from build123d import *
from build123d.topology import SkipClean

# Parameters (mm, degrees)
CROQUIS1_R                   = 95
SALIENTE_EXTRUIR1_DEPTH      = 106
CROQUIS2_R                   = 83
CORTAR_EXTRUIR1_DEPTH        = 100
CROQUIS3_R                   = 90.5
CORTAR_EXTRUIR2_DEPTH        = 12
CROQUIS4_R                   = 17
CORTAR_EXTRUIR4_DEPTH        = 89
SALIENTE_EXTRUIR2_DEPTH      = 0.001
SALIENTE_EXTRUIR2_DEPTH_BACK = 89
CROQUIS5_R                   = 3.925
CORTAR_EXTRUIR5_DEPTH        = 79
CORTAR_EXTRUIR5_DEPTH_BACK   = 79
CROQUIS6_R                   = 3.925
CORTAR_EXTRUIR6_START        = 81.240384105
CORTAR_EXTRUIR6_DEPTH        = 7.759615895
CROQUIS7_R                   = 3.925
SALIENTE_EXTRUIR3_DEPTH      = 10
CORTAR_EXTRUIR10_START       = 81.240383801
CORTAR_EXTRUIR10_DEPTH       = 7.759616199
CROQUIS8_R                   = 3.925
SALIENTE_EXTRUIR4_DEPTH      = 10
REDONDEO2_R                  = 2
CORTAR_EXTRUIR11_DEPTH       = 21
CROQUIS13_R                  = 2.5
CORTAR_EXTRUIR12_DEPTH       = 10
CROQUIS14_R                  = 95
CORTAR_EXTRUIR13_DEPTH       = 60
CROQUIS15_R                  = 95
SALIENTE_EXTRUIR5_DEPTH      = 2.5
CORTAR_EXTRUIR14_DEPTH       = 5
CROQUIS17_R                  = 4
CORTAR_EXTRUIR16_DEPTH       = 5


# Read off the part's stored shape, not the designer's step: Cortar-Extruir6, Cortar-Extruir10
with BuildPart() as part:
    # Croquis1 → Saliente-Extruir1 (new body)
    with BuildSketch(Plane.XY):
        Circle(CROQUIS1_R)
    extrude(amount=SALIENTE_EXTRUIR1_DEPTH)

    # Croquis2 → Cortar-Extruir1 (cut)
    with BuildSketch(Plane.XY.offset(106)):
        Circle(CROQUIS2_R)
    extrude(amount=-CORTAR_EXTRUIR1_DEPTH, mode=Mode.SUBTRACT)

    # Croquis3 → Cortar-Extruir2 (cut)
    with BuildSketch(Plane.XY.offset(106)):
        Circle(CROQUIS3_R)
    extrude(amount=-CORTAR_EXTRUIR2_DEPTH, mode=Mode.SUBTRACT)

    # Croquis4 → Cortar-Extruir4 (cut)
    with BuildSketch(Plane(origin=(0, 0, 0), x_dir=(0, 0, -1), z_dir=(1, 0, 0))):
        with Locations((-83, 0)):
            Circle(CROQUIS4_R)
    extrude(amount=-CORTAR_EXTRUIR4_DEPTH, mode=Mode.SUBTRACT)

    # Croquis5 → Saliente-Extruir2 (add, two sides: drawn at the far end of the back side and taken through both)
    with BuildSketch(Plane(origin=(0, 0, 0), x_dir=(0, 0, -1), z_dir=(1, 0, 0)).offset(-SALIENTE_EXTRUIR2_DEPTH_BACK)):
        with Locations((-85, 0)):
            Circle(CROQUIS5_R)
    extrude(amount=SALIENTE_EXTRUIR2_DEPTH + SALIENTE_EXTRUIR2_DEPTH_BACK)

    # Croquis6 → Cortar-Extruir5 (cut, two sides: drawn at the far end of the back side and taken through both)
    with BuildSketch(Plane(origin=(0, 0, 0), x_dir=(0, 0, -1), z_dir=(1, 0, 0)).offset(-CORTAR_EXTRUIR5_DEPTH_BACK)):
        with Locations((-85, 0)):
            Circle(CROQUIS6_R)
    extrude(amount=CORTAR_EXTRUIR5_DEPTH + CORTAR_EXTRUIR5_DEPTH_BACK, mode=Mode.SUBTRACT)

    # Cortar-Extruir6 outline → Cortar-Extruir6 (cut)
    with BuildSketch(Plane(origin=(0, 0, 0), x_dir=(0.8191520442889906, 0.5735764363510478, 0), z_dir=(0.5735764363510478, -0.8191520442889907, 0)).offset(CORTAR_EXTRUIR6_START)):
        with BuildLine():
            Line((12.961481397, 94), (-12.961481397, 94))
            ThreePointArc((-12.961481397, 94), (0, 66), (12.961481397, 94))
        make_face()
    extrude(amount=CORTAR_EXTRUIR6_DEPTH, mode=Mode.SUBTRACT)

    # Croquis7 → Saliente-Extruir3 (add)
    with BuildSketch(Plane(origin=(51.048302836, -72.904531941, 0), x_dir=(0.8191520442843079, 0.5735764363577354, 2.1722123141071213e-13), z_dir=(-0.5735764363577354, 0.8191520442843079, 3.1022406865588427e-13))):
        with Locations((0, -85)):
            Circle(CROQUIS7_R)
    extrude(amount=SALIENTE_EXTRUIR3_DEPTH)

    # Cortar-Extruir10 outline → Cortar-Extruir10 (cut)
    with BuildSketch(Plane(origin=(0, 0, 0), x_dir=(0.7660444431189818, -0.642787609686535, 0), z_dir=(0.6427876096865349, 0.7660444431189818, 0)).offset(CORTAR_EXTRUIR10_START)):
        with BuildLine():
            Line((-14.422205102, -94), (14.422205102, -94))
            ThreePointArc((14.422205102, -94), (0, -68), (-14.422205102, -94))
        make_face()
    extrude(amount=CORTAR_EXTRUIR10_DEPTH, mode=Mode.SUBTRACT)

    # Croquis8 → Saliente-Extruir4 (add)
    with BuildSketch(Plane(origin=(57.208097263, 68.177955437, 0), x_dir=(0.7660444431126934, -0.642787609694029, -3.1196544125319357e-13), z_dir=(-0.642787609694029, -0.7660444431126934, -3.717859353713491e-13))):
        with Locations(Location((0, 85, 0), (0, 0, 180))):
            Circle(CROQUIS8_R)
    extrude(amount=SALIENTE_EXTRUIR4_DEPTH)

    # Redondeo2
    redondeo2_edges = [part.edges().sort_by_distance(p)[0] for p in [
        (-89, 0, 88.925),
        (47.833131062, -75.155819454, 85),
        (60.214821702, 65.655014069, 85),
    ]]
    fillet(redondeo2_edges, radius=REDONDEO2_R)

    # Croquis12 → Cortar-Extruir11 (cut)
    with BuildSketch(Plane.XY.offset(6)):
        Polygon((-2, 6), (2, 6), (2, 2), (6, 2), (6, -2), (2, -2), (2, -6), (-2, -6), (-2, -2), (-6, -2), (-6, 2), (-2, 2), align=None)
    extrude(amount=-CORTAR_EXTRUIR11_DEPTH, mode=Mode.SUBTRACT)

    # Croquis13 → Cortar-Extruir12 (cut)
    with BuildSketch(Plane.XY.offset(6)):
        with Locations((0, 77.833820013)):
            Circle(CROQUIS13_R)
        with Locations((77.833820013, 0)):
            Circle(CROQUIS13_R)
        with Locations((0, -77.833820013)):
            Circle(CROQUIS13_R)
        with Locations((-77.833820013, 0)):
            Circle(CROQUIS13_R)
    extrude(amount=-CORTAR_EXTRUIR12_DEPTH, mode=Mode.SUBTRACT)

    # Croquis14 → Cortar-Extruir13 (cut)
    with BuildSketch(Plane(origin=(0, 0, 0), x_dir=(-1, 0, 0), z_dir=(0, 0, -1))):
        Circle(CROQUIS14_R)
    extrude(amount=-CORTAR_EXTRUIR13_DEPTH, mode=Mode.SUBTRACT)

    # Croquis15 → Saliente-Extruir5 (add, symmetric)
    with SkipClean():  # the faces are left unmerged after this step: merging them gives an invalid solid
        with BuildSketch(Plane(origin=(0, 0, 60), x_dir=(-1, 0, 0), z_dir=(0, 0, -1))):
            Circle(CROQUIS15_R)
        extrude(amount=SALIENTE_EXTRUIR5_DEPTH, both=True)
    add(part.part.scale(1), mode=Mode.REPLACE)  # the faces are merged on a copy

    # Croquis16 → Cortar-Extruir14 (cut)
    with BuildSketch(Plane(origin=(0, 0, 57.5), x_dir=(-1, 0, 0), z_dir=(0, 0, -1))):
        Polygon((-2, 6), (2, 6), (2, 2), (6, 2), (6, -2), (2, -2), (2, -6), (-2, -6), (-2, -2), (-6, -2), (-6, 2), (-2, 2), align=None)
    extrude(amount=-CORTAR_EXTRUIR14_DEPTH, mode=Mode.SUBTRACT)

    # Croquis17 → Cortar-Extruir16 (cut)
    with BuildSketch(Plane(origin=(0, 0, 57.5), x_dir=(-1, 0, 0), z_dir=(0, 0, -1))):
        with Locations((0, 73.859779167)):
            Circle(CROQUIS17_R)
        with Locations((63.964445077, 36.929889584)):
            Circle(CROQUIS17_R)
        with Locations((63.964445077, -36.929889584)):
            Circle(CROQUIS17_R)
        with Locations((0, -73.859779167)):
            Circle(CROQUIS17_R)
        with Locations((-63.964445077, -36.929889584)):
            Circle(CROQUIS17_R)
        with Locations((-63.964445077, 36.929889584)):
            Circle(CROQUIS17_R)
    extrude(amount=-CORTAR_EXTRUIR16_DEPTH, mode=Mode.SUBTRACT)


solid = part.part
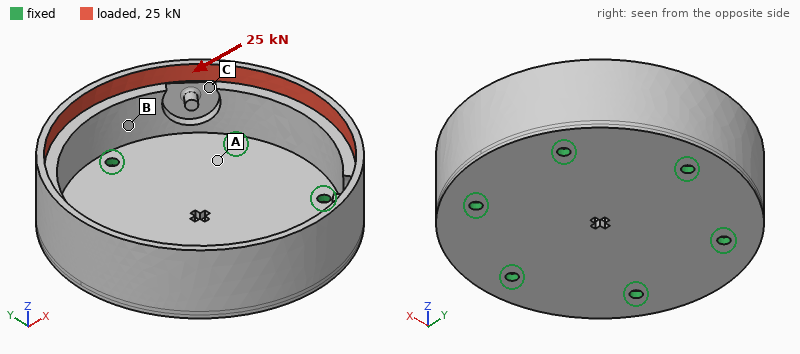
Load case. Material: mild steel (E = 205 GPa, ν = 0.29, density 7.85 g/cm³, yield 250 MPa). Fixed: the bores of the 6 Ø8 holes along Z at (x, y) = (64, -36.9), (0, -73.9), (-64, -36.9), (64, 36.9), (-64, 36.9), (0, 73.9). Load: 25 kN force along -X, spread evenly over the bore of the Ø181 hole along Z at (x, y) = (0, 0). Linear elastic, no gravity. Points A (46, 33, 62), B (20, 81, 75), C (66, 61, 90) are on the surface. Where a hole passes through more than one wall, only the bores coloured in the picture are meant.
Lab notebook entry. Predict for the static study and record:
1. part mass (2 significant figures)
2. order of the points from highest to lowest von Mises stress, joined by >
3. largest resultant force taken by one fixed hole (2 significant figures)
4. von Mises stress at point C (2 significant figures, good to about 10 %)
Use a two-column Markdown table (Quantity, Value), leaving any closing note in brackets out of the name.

| Quantity | Value |
|---|---|
| part mass | 2.9 kg |
| order of the points from highest to lowest von Mises stress, joined by > | C > B > A |
| largest resultant force taken by one fixed hole | 8.7 kN |
| von Mises stress at point C | 38 MPa |
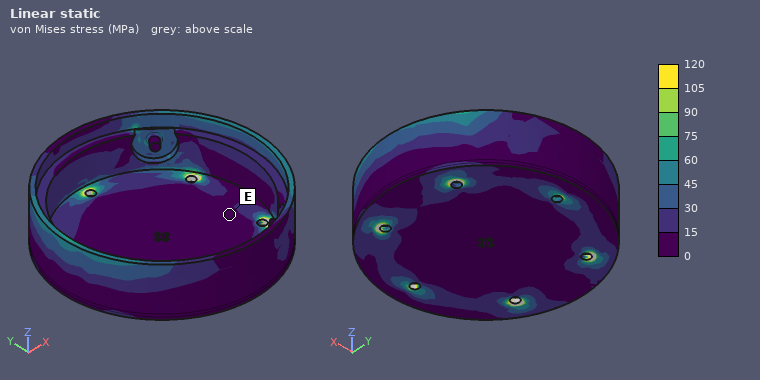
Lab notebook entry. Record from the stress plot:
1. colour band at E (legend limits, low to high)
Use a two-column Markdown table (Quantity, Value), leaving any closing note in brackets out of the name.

| Quantity | Value |
|---|---|
| colour band at E | 0 to 15 MPa |
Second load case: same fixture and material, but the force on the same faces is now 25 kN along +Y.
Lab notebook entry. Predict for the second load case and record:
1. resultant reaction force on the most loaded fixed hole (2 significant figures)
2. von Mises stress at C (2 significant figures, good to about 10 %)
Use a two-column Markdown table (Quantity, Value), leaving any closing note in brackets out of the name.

| Quantity | Value |
|---|---|
| resultant reaction force on the most loaded fixed hole | 8.0 kN |
| von Mises stress at C | 40 MPa |
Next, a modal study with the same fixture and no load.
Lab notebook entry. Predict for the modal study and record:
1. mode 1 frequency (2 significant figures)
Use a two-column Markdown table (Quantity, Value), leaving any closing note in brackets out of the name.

| Quantity | Value |
|---|---|
| mode 1 frequency | 2100 Hz |
